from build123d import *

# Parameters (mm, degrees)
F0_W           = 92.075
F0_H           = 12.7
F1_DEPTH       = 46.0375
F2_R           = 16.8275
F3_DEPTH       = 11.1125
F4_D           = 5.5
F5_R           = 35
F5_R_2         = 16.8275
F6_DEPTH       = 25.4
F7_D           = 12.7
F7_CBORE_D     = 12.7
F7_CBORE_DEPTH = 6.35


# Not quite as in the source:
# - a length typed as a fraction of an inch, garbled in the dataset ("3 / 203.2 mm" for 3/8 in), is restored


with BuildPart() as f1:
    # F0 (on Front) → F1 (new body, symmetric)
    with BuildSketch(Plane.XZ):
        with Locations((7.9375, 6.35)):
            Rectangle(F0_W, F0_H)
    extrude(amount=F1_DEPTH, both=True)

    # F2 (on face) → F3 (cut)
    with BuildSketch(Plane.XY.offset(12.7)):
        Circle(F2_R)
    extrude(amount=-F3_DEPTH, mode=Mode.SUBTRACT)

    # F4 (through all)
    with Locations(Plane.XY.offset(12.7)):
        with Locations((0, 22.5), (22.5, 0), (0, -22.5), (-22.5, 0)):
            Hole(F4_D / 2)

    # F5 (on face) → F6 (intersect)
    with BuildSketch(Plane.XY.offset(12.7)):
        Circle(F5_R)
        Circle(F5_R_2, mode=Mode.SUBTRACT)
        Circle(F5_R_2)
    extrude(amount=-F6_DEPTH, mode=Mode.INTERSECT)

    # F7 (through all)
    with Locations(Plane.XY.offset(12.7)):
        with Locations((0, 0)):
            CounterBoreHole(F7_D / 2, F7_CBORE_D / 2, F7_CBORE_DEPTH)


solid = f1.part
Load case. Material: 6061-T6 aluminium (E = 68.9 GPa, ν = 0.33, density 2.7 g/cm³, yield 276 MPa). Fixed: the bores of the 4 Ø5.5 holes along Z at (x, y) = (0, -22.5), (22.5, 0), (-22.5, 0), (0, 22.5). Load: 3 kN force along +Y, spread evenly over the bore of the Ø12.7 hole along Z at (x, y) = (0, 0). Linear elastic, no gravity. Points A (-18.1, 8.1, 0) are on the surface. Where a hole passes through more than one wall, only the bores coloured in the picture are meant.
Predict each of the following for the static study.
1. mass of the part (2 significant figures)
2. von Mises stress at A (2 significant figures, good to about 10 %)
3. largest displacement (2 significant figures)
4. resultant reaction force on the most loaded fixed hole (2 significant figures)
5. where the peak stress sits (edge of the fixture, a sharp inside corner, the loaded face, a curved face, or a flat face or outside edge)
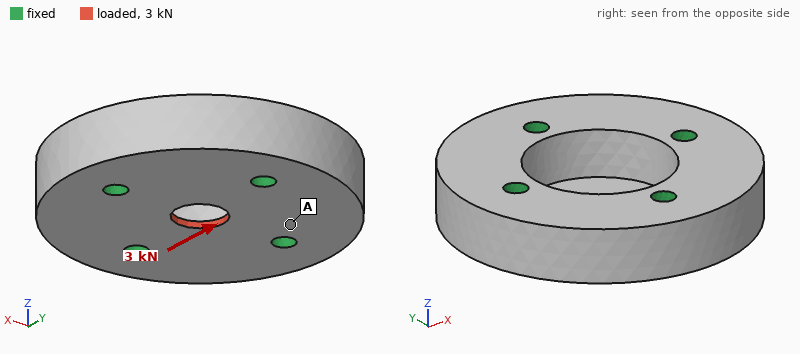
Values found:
100 g
8.5 MPa
9.3 µm
880 N
the loaded face
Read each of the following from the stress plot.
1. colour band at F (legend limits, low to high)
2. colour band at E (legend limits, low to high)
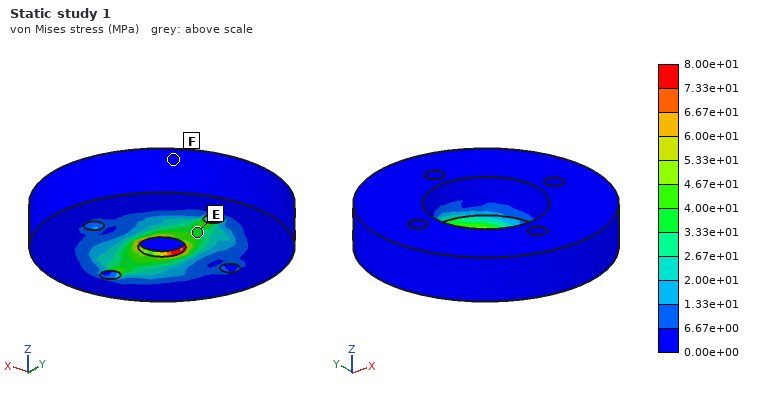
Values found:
0.00e+00 to 6.67e+00 MPa
3.33e+01 to 4.00e+01 MPa
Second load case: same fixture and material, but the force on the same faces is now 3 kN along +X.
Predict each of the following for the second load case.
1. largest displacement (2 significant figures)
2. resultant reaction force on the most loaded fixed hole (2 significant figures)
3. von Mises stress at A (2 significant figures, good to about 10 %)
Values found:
9.3 µm
880 N
16 MPa
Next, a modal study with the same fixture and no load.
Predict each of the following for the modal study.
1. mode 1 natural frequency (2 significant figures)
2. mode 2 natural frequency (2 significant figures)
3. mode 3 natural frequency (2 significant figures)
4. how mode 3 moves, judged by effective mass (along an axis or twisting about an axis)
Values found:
15 kHz
20 kHz
22 kHz
twisting about Y
